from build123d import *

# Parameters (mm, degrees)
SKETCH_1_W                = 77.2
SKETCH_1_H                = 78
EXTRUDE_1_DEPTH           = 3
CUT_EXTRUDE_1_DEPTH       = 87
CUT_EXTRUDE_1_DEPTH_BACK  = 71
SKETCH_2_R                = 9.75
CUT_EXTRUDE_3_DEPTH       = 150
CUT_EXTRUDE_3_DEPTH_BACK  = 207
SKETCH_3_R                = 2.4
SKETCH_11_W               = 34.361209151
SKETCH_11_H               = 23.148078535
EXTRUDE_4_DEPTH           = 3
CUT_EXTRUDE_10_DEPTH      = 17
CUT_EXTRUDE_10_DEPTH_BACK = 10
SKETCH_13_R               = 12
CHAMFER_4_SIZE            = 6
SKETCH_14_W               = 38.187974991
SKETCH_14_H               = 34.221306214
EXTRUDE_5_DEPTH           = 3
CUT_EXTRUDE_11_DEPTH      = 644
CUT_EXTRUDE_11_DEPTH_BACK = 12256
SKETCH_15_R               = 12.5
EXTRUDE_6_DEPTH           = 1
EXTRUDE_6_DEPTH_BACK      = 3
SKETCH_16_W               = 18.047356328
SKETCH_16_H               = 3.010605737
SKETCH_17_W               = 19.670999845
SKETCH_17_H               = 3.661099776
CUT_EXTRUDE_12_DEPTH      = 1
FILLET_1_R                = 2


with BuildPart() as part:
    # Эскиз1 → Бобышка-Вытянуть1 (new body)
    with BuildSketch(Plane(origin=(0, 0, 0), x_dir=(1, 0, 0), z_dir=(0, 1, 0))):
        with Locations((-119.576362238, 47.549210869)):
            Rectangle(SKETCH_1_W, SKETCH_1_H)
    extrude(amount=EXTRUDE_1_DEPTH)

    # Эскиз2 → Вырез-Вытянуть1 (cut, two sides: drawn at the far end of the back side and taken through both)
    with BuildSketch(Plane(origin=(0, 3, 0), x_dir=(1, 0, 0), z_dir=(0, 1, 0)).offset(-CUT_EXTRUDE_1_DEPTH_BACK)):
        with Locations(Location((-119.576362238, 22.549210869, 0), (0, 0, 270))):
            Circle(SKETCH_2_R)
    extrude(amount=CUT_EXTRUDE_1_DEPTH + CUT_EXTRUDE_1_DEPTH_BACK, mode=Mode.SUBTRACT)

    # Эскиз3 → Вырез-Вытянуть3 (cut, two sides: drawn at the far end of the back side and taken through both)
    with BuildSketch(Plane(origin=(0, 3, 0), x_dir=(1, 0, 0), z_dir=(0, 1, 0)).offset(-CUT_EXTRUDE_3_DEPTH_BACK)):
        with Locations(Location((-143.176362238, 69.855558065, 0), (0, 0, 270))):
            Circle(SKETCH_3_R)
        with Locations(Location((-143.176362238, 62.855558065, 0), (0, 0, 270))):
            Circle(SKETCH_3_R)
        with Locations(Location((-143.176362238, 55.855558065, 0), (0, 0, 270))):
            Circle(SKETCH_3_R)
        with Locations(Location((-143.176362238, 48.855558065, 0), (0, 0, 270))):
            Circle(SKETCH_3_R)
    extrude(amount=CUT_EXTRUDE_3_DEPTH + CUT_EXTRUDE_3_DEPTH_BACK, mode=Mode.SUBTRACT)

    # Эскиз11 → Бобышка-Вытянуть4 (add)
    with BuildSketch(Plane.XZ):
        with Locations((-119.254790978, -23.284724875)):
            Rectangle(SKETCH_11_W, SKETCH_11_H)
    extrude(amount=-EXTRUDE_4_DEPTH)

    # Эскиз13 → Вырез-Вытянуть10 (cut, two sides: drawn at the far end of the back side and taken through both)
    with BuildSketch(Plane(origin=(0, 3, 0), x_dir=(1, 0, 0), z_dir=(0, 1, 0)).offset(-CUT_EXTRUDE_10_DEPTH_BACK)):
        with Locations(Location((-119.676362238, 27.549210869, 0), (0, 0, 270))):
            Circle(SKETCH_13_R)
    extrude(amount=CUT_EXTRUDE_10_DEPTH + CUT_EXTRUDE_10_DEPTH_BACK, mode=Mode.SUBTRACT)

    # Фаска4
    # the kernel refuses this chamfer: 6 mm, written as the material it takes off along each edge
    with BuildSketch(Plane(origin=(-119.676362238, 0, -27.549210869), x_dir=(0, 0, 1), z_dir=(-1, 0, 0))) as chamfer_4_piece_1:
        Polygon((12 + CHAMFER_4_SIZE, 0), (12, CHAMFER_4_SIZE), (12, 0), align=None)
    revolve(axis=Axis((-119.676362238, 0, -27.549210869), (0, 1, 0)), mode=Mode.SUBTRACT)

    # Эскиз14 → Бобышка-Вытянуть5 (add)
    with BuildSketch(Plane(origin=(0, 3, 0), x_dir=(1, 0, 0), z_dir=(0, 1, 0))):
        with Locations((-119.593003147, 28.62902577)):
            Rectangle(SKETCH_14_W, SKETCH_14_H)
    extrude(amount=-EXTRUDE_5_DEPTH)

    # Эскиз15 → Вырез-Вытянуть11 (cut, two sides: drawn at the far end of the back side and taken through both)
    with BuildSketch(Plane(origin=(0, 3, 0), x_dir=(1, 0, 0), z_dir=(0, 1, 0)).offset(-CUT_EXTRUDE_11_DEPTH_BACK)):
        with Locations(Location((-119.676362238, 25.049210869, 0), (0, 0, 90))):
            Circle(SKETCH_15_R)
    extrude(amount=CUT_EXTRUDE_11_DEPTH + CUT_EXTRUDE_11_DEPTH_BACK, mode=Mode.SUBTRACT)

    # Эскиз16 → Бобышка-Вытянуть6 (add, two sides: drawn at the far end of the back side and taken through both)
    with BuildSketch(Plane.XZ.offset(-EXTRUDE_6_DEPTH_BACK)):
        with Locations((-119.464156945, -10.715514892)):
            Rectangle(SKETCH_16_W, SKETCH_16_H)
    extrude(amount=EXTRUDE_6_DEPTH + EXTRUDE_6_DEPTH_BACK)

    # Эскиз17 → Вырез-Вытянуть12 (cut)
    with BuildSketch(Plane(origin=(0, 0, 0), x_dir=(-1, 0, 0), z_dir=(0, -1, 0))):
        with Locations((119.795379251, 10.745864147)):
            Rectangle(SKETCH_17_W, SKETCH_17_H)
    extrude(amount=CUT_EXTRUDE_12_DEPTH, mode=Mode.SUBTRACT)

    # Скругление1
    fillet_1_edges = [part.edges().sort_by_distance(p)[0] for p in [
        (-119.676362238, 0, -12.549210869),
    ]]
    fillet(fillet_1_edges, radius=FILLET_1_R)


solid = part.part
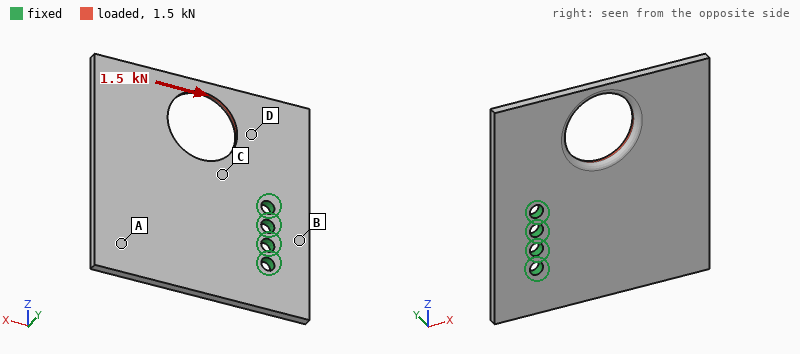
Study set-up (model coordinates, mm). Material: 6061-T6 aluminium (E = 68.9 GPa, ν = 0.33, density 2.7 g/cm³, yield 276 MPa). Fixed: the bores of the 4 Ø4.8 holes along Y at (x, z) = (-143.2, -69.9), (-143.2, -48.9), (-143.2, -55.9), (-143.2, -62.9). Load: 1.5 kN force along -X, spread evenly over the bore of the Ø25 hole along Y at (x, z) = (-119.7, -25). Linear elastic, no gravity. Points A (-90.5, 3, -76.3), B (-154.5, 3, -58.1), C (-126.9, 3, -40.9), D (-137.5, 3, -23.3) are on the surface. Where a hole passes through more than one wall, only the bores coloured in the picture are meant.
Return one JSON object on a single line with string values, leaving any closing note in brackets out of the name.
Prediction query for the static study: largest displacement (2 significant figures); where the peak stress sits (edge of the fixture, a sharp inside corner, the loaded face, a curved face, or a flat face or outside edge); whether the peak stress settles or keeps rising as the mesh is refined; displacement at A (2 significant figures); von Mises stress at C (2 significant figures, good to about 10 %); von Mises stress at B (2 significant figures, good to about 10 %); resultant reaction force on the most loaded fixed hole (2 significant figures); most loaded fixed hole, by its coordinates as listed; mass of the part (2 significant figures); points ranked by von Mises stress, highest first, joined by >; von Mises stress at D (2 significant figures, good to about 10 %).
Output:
{"largest displacement": "0.30 mm", "where the peak stress sits": "edge of the fixture", "whether the peak stress settles or keeps rising as the mesh is refined": "keeps rising", "displacement at A": "0.11 mm", "von Mises stress at C": "45 MPa", "von Mises stress at B": "17 MPa", "resultant reaction force on the most loaded fixed hole": "2.5 kN", "most loaded fixed hole, by its coordinates as listed": "(-143.2, -48.9)", "mass of the part": "44 g", "points ranked by von Mises stress, highest first, joined by >": "C > D > B > A", "von Mises stress at D": "29 MPa"}
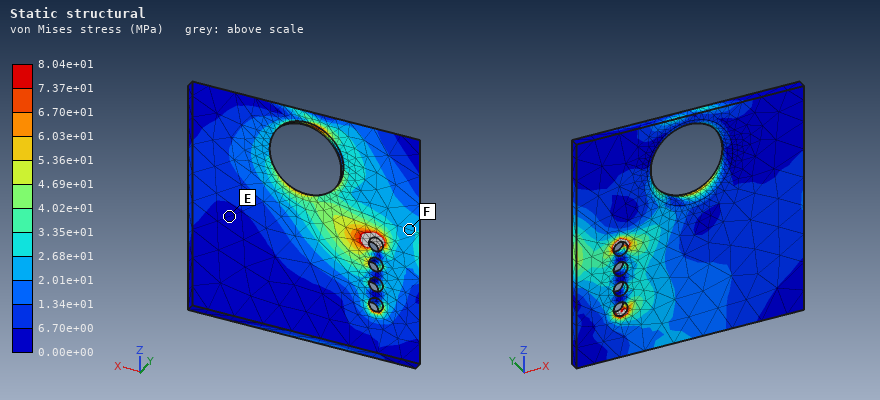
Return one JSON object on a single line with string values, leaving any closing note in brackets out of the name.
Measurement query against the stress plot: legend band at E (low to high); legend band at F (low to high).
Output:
{"legend band at E": "0.00e+00 to 6.70e+00 MPa", "legend band at F": "2.01e+01 to 2.68e+01 MPa"}
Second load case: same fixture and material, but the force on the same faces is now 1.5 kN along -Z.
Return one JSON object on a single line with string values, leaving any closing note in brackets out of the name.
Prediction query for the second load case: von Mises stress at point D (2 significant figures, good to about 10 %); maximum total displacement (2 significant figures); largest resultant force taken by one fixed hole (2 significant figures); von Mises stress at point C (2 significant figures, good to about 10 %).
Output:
{"von Mises stress at point D": "24 MPa", "maximum total displacement": "0.17 mm", "largest resultant force taken by one fixed hole": "1.5 kN", "von Mises stress at point C": "26 MPa"}
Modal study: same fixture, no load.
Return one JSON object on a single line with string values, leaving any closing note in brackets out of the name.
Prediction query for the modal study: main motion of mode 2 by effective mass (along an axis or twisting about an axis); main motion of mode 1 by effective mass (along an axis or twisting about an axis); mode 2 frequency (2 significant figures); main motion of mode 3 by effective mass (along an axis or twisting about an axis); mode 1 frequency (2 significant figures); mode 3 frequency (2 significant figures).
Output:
{"main motion of mode 2 by effective mass": "twisting about X", "main motion of mode 1 by effective mass": "along Y", "mode 2 frequency": "1000 Hz", "main motion of mode 3 by effective mass": "along Y", "mode 1 frequency": "550 Hz", "mode 3 frequency": "1800 Hz"}
